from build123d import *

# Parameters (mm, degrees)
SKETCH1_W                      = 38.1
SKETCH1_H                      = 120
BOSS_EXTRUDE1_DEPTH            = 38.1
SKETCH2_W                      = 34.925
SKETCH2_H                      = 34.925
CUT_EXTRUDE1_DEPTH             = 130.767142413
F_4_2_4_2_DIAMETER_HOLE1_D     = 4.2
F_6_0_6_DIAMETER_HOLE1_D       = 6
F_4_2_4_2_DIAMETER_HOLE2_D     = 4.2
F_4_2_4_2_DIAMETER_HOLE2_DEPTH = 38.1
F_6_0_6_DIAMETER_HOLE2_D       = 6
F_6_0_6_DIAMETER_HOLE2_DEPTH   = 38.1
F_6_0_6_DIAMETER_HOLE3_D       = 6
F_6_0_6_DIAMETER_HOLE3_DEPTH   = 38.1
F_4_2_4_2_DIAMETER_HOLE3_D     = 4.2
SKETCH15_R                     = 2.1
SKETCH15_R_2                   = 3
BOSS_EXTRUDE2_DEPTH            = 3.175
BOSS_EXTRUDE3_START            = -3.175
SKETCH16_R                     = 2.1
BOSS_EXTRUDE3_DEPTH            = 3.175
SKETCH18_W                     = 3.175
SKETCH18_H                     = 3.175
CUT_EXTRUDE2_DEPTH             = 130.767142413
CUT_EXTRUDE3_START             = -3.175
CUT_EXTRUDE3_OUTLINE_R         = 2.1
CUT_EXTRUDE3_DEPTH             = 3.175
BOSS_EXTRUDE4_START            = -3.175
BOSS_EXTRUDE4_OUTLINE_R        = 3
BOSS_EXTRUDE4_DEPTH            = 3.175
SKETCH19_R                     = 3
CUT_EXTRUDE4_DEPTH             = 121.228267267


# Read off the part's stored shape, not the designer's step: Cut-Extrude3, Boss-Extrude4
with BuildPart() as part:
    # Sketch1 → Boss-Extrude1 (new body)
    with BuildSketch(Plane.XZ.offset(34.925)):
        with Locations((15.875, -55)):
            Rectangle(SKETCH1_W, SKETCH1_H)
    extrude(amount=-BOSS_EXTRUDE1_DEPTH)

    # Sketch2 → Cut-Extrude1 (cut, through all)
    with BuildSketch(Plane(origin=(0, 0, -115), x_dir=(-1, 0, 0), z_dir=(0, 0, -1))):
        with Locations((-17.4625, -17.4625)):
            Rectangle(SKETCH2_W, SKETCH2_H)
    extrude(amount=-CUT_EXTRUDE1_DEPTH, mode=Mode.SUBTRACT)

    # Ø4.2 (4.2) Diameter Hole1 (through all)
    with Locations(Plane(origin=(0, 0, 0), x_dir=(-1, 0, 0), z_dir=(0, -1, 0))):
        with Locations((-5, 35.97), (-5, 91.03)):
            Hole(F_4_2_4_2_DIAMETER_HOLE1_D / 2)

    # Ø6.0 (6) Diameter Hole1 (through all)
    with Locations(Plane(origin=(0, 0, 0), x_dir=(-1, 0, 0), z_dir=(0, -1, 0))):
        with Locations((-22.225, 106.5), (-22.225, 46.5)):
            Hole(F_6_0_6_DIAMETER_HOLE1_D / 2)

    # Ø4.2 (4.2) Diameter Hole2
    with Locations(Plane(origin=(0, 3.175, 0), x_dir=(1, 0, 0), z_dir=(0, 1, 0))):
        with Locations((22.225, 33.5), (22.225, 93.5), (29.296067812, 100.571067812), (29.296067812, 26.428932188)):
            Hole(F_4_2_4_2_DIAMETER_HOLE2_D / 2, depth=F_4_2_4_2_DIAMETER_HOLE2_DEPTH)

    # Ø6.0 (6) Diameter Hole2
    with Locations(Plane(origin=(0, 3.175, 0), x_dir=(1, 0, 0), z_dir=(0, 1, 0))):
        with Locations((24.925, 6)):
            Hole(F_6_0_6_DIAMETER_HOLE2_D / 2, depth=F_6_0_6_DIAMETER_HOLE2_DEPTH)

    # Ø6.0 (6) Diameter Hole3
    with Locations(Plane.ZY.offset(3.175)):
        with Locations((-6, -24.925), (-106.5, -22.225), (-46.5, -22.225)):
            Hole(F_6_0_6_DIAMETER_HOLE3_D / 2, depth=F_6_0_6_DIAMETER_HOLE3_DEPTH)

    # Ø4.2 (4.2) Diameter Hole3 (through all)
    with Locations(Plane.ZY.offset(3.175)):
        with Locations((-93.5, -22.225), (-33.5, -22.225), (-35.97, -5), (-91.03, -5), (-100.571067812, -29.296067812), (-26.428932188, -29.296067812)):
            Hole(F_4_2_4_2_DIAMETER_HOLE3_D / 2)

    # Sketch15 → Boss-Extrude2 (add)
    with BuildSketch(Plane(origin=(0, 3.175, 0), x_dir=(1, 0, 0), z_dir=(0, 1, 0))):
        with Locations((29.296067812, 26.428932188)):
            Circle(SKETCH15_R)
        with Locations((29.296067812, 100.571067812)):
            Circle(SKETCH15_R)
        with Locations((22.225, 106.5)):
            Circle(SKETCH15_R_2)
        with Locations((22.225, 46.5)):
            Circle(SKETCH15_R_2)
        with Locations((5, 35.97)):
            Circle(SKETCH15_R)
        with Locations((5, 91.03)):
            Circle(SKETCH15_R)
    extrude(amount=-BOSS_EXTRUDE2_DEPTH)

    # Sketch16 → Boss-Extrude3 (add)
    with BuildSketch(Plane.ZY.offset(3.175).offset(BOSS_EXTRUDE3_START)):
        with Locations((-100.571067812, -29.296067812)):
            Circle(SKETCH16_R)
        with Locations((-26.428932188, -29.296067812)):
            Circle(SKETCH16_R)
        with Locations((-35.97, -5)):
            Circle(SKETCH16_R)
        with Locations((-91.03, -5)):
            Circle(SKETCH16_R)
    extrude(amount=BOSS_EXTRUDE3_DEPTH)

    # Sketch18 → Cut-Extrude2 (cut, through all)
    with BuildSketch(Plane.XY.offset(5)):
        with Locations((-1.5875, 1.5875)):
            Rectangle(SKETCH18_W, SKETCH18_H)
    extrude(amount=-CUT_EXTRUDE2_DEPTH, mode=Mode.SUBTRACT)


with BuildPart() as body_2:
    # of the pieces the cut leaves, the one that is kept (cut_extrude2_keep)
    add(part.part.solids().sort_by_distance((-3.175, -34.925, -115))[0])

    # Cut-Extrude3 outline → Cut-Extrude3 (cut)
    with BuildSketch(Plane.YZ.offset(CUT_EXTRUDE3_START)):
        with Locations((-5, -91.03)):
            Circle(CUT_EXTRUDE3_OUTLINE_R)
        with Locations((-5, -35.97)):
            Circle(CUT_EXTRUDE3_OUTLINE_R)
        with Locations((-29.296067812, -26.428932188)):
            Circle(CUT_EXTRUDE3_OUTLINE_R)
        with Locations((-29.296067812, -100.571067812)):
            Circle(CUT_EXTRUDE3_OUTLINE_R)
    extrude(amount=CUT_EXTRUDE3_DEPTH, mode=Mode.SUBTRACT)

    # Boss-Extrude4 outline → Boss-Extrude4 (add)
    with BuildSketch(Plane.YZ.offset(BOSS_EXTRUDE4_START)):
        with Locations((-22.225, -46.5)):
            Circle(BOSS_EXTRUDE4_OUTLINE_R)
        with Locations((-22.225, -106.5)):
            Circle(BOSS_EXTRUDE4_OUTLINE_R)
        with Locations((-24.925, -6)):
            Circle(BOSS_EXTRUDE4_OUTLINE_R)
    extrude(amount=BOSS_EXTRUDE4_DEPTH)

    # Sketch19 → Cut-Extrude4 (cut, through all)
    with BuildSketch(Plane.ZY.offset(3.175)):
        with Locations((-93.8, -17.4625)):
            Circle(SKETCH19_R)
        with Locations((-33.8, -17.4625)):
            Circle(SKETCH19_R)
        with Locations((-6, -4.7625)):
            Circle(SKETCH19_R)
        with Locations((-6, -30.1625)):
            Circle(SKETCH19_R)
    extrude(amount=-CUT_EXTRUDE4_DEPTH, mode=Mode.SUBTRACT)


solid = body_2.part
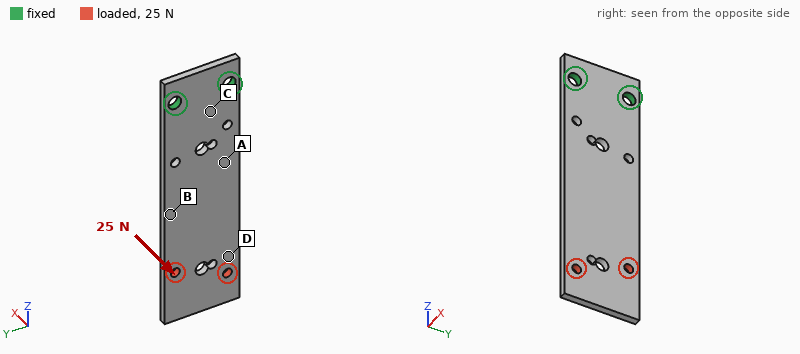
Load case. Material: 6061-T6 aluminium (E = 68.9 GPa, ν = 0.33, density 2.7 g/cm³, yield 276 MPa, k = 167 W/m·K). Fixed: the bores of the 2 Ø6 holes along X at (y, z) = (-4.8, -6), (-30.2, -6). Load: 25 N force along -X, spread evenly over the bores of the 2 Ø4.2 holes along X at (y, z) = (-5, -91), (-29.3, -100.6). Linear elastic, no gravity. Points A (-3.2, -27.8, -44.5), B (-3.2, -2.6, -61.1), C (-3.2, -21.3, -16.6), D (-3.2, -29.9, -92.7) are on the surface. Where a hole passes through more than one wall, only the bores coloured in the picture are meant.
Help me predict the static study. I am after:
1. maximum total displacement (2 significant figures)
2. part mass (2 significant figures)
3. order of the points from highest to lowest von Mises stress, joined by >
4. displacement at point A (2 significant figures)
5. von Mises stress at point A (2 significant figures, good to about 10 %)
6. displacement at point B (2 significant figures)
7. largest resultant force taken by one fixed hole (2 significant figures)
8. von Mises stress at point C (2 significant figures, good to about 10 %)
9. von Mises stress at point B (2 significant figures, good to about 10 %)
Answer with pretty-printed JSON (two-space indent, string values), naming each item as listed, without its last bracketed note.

{
  "maximum total displacement": "1.3 mm",
  "part mass": "34 g",
  "order of the points from highest to lowest von Mises stress, joined by >": "C > A > B > D",
  "displacement at point A": "0.22 mm",
  "von Mises stress at point A": "22 MPa",
  "displacement at point B": "0.43 mm",
  "largest resultant force taken by one fixed hole": "13 N",
  "von Mises stress at point C": "30 MPa",
  "von Mises stress at point B": "15 MPa"
}
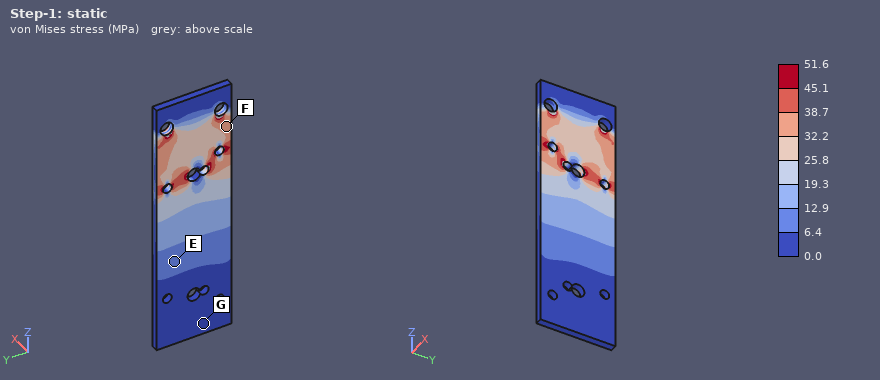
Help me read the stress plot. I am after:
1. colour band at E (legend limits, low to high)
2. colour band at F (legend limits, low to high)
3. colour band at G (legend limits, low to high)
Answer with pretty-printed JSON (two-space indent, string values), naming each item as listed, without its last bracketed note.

{
  "colour band at E": "6.4 to 12.9 MPa",
  "colour band at F": "32.2 to 38.7 MPa",
  "colour band at G": "0.0 to 6.4 MPa"
}
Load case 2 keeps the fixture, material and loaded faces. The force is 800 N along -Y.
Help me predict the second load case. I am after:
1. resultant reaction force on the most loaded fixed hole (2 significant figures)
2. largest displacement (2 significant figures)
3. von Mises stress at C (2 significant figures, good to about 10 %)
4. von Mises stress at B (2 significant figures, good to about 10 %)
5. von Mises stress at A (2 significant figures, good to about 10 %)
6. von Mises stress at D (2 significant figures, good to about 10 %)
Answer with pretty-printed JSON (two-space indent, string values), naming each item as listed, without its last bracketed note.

{
  "resultant reaction force on the most loaded fixed hole": "2.7 kN",
  "largest displacement": "0.38 mm",
  "von Mises stress at C": "26 MPa",
  "von Mises stress at B": "36 MPa",
  "von Mises stress at A": "42 MPa",
  "von Mises stress at D": "16 MPa"
}
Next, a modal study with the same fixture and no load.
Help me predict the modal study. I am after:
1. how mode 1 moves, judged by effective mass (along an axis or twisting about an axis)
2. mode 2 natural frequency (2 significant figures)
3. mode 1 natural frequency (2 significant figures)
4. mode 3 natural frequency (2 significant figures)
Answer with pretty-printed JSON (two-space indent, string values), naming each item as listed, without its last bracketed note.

{
  "how mode 1 moves, judged by effective mass": "along X",
  "mode 2 natural frequency": "1400 Hz",
  "mode 1 natural frequency": "220 Hz",
  "mode 3 natural frequency": "1400 Hz"
}
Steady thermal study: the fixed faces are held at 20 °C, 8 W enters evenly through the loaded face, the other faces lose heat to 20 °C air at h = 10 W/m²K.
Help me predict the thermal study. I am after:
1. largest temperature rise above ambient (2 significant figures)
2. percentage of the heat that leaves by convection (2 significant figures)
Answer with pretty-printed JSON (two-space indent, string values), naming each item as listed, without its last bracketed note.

{
  "largest temperature rise above ambient": "38 K",
  "percentage of the heat that leaves by convection": "21 %"
}
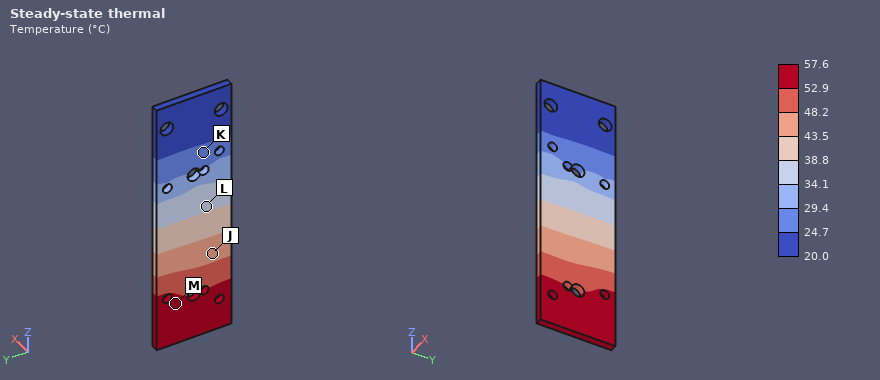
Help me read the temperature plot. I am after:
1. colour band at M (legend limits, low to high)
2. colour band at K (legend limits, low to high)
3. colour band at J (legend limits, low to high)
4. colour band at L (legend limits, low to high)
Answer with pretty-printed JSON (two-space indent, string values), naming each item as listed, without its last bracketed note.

{
  "colour band at M": "52.9 to 57.6 °C",
  "colour band at K": "24.7 to 29.4 °C",
  "colour band at J": "43.5 to 48.2 °C",
  "colour band at L": "34.1 to 38.8 °C"
}
